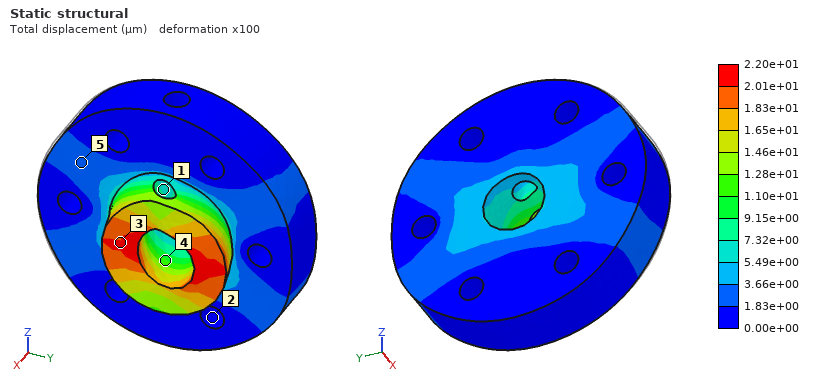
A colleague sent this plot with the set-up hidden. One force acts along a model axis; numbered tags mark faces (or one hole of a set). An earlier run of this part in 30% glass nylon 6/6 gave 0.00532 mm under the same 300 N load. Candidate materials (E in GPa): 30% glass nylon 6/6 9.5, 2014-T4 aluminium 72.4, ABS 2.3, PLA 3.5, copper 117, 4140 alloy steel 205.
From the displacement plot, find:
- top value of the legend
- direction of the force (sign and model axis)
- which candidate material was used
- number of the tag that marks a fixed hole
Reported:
2.20e+01 µm
+Y
ABS
2
